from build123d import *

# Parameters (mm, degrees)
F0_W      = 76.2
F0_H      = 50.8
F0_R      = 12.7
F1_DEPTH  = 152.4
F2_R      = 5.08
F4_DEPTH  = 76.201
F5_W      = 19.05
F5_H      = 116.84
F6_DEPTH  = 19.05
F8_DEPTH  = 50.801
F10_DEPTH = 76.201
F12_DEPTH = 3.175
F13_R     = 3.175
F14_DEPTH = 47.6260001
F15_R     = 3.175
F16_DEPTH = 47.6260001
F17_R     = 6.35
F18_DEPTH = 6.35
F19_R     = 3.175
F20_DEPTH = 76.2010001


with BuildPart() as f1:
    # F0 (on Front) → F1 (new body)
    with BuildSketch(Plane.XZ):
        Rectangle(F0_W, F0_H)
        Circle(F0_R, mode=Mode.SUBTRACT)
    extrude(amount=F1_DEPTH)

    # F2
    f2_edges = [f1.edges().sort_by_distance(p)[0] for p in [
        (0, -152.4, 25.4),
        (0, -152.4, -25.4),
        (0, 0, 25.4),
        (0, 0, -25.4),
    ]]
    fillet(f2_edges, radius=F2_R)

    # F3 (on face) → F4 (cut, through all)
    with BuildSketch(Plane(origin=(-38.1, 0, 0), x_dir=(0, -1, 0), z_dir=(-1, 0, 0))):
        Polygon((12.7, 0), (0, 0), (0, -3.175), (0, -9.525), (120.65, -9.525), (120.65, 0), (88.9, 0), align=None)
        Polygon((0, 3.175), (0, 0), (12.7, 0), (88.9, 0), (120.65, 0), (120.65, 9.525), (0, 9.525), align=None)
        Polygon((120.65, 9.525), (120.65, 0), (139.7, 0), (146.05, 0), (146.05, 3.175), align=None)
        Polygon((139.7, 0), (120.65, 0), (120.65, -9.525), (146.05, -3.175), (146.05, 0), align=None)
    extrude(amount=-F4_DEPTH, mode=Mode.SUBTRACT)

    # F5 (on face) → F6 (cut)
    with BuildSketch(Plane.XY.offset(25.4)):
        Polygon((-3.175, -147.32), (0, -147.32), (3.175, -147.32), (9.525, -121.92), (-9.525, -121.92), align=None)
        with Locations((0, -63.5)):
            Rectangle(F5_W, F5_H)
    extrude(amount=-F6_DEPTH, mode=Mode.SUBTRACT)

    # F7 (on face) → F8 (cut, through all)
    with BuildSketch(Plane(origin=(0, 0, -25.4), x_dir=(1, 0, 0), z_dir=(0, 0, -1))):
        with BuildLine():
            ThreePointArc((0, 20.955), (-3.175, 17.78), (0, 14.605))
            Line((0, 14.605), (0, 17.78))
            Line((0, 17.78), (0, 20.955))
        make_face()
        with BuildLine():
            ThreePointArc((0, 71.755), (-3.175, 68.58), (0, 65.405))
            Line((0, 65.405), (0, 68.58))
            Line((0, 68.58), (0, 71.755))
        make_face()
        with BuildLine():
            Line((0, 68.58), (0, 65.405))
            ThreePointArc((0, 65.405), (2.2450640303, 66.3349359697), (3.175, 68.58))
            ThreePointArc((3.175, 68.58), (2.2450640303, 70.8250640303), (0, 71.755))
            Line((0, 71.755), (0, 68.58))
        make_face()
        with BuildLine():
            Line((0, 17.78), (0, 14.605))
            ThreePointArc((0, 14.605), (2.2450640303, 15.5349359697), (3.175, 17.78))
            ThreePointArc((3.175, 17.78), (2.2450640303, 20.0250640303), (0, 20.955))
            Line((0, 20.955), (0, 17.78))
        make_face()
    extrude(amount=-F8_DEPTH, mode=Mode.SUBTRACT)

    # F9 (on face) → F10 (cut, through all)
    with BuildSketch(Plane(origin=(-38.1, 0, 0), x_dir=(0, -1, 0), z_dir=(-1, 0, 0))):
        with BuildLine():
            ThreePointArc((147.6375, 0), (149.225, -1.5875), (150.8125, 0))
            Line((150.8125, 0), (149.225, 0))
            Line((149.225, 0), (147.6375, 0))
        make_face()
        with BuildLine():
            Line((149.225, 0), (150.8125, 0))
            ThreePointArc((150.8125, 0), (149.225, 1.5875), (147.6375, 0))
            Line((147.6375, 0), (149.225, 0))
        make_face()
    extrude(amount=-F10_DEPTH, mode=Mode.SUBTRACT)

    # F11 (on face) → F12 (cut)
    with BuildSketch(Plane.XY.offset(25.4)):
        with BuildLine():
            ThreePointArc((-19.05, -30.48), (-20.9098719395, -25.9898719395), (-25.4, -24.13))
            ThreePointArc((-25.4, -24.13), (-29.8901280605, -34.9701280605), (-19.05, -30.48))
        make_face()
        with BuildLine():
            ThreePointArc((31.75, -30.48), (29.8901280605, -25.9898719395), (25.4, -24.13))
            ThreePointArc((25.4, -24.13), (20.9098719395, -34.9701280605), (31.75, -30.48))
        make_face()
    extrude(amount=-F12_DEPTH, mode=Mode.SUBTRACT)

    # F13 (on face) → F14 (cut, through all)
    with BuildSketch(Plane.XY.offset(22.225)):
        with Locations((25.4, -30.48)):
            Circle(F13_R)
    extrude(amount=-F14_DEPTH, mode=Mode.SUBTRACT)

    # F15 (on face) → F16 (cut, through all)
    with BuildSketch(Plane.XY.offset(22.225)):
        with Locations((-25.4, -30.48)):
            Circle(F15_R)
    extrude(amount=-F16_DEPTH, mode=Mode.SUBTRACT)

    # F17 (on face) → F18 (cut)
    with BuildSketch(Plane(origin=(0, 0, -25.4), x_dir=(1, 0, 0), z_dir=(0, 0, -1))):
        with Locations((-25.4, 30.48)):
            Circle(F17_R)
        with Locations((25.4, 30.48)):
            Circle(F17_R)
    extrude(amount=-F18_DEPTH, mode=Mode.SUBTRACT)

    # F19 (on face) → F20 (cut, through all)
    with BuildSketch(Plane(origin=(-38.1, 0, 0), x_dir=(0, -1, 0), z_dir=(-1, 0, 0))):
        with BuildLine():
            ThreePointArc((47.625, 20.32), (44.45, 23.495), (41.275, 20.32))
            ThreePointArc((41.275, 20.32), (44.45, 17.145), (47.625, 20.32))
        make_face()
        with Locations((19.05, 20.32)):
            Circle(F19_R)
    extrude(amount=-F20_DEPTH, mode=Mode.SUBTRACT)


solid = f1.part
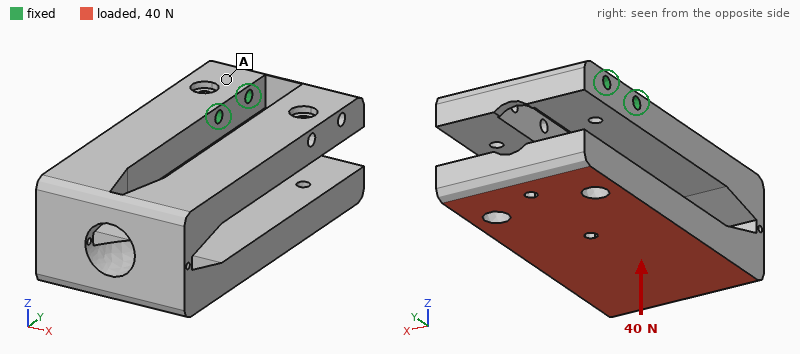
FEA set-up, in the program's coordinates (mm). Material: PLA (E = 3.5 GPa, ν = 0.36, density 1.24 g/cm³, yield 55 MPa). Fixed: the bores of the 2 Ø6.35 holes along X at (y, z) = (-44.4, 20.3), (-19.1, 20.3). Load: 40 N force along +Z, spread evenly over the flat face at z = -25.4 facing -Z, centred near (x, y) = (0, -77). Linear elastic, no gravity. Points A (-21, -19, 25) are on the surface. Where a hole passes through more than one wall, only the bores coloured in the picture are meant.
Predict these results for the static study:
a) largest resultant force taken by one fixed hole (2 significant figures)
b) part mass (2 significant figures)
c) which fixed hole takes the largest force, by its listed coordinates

67 N
410 g
(-44.4, 20.3)
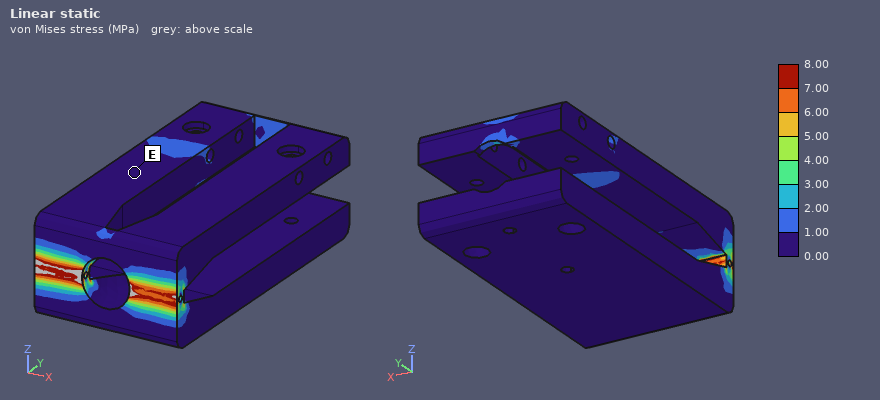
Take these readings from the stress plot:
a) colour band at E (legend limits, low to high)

0.00 to 1.00 MPa
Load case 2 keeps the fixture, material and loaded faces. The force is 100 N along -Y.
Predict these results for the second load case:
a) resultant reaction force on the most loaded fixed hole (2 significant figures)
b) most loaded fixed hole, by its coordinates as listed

130 N
(-19.1, 20.3)
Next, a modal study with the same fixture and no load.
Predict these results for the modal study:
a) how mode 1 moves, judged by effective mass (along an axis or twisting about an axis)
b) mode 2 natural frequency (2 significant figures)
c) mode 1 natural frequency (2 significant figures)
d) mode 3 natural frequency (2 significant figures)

along Z
100 Hz
61 Hz
130 Hz
